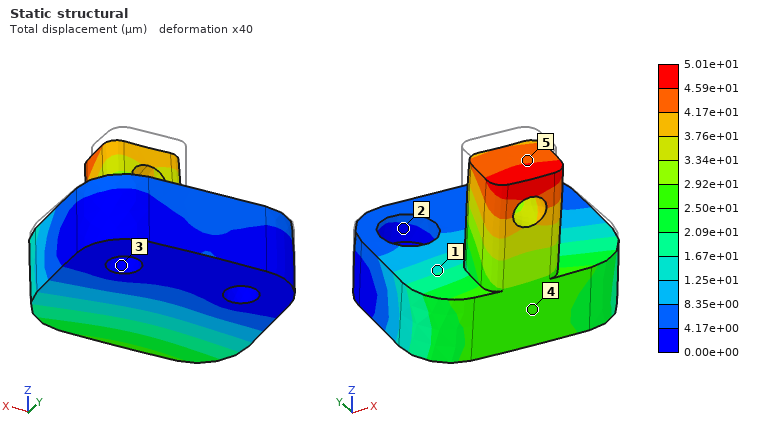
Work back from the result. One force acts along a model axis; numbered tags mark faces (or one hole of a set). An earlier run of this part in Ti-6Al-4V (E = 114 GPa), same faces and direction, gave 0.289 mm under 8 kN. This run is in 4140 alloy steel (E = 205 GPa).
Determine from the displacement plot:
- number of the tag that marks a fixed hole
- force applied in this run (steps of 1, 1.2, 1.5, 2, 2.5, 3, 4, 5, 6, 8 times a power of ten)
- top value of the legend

3
2.5 kN
5.01e+01 µm
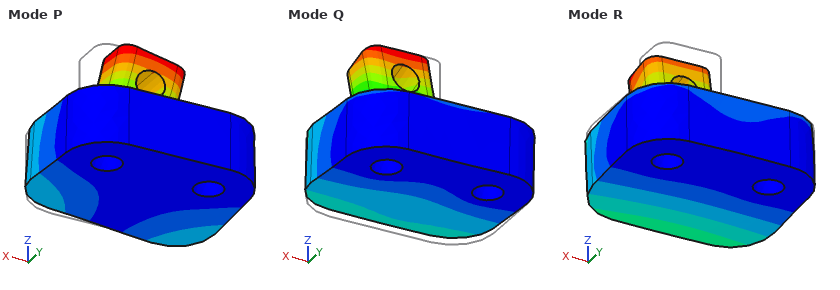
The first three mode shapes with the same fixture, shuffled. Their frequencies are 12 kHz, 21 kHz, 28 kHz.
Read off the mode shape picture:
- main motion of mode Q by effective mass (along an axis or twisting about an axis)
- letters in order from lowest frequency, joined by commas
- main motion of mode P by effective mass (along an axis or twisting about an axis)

along Z
R, P, Q
along X
